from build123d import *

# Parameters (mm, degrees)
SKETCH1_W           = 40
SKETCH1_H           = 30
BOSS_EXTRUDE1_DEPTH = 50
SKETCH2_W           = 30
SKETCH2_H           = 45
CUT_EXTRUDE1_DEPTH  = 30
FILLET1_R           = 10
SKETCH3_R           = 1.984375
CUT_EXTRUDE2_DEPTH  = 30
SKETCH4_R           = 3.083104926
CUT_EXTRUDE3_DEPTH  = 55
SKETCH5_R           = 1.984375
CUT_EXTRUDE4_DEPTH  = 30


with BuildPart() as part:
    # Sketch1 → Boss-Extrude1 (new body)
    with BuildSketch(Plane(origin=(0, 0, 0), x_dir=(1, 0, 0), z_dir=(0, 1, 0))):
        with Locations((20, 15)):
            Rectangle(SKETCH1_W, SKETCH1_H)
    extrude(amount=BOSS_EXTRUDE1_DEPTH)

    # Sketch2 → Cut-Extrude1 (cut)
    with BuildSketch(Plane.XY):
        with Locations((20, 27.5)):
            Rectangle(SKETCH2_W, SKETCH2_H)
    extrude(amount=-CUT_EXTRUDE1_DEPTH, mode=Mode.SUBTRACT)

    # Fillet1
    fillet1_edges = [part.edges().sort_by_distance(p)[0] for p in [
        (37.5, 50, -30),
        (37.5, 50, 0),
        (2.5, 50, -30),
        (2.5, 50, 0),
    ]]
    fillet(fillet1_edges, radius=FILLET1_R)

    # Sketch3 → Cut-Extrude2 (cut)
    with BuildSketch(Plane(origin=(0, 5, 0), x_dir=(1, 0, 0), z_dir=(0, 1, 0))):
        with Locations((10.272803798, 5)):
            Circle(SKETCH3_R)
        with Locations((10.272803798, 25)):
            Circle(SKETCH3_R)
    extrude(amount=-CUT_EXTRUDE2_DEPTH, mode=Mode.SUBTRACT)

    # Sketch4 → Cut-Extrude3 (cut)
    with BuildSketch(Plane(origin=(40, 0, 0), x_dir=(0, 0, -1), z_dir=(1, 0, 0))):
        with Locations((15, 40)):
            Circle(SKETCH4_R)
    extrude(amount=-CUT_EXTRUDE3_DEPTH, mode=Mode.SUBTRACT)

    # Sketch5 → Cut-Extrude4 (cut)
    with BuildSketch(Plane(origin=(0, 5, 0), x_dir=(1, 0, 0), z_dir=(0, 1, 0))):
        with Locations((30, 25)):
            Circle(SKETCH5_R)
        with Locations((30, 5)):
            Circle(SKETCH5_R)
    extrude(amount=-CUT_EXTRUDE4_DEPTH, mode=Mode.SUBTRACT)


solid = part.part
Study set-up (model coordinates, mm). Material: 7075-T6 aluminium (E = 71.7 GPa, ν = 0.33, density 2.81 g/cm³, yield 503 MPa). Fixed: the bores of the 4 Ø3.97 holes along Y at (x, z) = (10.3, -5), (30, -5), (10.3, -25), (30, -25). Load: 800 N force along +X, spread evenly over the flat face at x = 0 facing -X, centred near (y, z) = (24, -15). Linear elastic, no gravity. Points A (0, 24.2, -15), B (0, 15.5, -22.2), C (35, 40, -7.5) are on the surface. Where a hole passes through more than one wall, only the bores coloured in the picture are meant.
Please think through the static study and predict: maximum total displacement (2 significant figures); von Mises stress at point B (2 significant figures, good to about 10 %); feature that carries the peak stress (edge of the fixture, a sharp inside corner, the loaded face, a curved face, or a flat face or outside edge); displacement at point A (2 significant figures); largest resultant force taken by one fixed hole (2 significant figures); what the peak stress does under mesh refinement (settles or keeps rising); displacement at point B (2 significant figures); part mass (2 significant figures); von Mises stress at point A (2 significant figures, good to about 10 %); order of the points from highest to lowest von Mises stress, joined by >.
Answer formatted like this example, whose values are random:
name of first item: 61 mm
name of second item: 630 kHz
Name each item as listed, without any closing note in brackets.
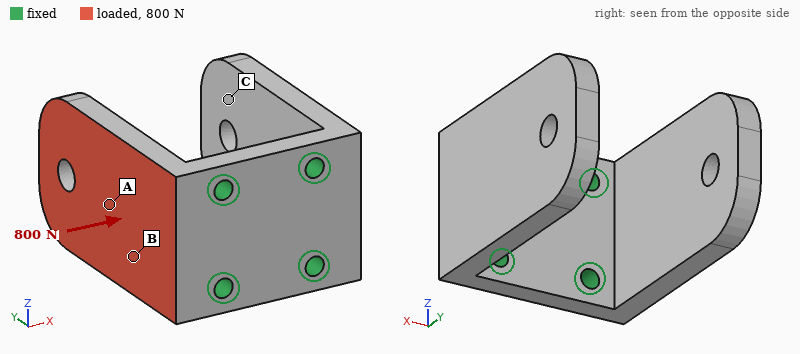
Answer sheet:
maximum total displacement: 0.62 mm
von Mises stress at point B: 66 MPa
feature that carries the peak stress: edge of the fixture
displacement at point A: 0.23 mm
largest resultant force taken by one fixed hole: 370 N
what the peak stress does under mesh refinement: keeps rising
displacement at point B: 0.12 mm
part mass: 52 g
von Mises stress at point A: 35 MPa
order of the points from highest to lowest von Mises stress, joined by >: B > A > C
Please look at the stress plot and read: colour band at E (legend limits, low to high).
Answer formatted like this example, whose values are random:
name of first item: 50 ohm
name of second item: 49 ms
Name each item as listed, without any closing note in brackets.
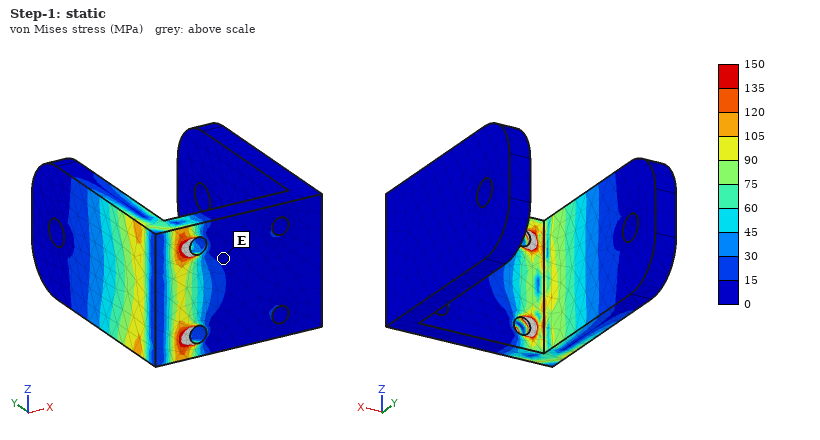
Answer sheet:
colour band at E: 0 to 15 MPa
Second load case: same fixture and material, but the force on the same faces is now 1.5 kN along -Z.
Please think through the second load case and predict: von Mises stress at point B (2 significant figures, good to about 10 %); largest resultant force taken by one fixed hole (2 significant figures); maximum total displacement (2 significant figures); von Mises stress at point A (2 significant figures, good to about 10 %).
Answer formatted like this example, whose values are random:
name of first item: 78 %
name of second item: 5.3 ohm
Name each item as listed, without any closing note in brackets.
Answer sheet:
von Mises stress at point B: 21 MPa
largest resultant force taken by one fixed hole: 1.8 kN
maximum total displacement: 97 µm
von Mises stress at point A: 24 MPa
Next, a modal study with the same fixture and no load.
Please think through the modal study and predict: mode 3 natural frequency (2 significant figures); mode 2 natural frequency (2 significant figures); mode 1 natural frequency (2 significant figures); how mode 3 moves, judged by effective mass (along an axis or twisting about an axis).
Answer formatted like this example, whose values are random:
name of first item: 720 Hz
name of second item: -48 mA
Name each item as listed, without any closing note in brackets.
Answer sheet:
mode 3 natural frequency: 4900 Hz
mode 2 natural frequency: 1600 Hz
mode 1 natural frequency: 1600 Hz
how mode 3 moves, judged by effective mass: along Z
